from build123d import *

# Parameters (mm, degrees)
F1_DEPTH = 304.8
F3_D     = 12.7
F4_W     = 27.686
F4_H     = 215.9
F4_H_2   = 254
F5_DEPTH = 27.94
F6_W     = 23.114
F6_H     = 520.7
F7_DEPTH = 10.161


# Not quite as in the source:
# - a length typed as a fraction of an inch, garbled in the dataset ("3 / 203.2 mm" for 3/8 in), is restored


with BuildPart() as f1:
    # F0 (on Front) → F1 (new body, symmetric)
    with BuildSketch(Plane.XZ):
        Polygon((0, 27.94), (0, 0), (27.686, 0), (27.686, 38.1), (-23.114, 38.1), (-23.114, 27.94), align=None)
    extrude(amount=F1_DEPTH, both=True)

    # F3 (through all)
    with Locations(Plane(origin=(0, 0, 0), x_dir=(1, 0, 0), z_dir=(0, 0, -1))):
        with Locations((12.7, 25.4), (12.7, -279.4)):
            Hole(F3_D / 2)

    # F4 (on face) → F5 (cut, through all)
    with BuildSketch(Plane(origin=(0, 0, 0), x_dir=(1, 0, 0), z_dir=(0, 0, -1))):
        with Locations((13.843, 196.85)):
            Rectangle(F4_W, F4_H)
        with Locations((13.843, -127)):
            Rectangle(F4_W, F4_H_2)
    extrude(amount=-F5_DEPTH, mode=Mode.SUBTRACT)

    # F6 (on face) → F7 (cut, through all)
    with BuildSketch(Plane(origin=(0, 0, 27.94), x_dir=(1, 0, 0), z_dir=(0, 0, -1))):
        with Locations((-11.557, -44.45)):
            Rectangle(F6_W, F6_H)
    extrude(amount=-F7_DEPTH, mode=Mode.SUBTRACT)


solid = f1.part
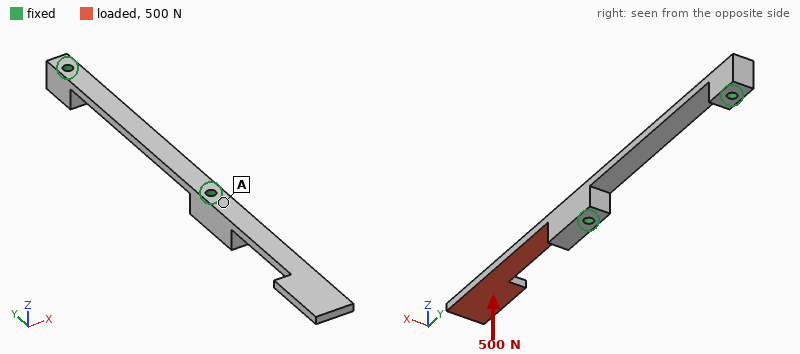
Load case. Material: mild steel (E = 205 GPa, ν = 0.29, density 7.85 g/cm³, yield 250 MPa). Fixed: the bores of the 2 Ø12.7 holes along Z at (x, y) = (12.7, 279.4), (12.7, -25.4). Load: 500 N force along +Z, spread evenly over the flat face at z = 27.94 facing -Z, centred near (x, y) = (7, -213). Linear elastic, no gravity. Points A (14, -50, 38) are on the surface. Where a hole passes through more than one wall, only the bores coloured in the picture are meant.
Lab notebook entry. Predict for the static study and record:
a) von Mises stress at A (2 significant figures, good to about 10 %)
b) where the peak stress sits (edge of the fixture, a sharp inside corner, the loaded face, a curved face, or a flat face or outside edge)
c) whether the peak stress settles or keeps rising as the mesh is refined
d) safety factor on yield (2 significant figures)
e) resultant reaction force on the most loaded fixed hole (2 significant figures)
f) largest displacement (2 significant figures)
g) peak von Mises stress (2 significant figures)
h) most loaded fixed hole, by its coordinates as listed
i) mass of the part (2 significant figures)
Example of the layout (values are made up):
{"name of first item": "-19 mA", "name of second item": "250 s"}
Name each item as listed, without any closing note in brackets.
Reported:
{"von Mises stress at A": "13 MPa", "where the peak stress sits": "a flat face or outside edge", "whether the peak stress settles or keeps rising as the mesh is refined": "settles", "safety factor on yield": "2.0", "resultant reaction force on the most loaded fixed hole": "500 N", "largest displacement": "1.8 mm", "peak von Mises stress": "120 MPa", "most loaded fixed hole, by its coordinates as listed": "(12.7, -25.4)", "mass of the part": "2.3 kg"}
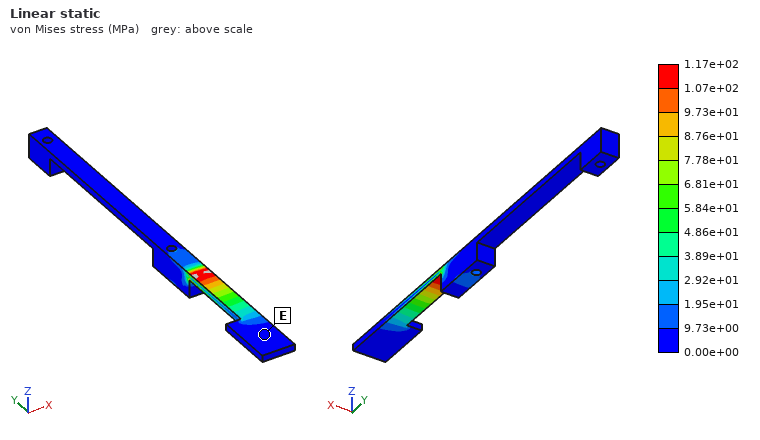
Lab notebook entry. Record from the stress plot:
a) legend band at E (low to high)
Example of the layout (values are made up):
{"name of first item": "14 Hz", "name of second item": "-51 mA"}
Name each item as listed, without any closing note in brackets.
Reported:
{"legend band at E": "0.00e+00 to 9.73e+00 MPa"}
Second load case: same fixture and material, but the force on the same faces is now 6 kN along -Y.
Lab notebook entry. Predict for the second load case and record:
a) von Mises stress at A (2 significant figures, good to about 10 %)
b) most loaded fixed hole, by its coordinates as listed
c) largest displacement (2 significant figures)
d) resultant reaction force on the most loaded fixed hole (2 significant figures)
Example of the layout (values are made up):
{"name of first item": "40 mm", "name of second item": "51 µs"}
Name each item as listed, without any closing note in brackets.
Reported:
{"von Mises stress at A": "14 MPa", "most loaded fixed hole, by its coordinates as listed": "(12.7, -25.4)", "largest displacement": "1.1 mm", "resultant reaction force on the most loaded fixed hole": "6.0 kN"}
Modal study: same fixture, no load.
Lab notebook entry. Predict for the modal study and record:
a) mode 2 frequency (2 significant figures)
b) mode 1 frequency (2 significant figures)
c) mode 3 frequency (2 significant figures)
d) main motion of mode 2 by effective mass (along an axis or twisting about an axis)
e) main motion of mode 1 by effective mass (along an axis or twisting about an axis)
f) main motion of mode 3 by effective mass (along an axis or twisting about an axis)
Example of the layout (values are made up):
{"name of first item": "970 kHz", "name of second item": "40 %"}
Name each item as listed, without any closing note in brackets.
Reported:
{"mode 2 frequency": "290 Hz", "mode 1 frequency": "130 Hz", "mode 3 frequency": "750 Hz", "main motion of mode 2 by effective mass": "along X", "main motion of mode 1 by effective mass": "along Z", "main motion of mode 3 by effective mass": "along Z"}
